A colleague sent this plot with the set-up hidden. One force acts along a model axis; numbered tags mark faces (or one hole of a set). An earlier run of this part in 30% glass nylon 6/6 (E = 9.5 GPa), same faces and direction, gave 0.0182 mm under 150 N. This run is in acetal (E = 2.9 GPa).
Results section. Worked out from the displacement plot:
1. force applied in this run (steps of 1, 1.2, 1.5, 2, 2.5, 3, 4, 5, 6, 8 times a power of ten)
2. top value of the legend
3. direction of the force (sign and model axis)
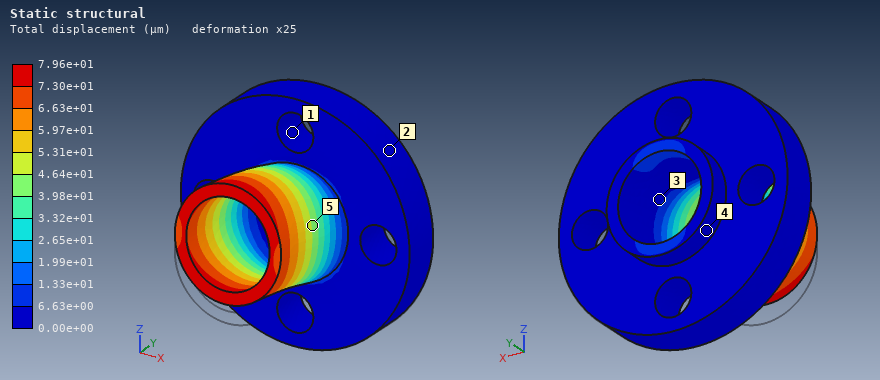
200 N
7.96e+01 µm
+Z
